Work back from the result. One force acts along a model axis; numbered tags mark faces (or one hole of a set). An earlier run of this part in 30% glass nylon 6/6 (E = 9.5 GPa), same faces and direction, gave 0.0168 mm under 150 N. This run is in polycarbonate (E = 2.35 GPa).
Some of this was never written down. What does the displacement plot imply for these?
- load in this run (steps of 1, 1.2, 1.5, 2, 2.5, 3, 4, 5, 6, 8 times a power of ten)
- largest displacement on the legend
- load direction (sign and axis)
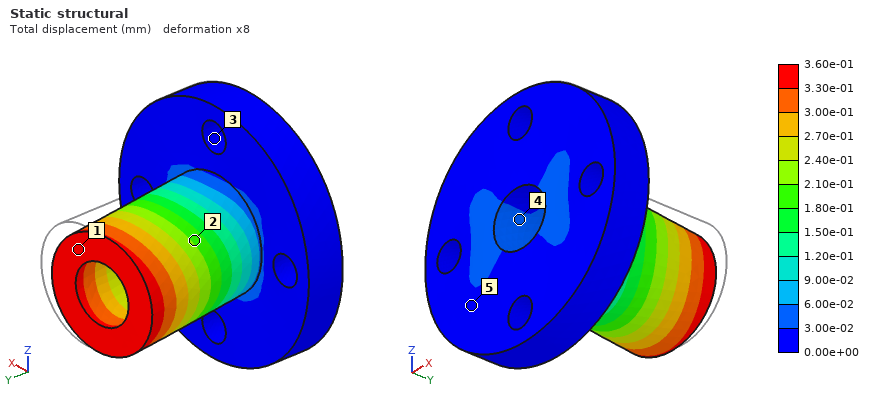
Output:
800 N
3.60e-01 mm
-X
